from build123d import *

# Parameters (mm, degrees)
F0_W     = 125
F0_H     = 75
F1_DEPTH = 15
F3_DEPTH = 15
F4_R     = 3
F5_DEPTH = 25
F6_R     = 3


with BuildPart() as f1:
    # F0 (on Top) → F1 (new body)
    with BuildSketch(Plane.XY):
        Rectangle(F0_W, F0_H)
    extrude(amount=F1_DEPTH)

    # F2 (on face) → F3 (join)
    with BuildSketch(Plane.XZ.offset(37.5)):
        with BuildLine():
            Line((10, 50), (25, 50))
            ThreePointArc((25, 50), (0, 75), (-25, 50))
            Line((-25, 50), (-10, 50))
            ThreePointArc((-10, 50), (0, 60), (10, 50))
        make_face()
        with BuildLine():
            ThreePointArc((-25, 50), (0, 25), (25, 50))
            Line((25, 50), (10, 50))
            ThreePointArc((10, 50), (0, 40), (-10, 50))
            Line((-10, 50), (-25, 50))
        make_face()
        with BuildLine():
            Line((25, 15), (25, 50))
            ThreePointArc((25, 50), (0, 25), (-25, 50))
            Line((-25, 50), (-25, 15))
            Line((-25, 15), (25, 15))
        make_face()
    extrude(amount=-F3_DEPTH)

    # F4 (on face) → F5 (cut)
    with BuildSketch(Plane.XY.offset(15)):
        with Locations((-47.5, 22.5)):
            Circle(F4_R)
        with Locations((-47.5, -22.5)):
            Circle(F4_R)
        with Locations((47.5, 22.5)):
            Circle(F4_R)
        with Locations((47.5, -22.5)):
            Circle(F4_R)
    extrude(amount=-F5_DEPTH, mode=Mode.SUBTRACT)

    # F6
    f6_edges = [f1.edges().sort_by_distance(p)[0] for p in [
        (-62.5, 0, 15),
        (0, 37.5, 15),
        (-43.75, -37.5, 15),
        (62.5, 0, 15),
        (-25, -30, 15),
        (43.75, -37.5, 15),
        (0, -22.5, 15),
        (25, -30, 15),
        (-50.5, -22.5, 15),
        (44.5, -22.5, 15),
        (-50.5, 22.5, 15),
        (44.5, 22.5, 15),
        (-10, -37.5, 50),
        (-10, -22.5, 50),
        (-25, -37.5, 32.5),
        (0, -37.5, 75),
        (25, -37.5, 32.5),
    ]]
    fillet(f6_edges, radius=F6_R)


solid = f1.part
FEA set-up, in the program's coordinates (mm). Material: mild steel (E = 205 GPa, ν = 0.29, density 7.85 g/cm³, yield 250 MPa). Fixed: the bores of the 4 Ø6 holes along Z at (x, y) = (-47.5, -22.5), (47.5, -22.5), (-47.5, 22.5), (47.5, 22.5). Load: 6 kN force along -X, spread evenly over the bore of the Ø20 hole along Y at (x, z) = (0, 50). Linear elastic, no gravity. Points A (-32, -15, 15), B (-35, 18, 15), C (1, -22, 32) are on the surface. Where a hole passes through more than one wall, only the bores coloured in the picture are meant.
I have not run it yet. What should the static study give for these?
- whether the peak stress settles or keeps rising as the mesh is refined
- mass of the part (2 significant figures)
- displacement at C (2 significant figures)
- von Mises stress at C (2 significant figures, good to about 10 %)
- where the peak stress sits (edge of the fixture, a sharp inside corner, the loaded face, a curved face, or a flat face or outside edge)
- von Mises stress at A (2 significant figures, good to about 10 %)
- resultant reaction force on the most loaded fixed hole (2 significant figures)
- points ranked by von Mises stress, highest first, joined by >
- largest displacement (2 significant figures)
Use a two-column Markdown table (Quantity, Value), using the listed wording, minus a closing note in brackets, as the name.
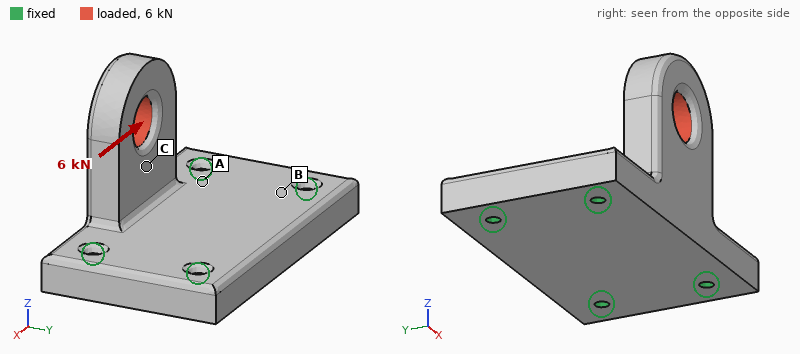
| Quantity | Value |
|---|---|
| whether the peak stress settles or keeps rising as the mesh is refined | keeps rising |
| mass of the part | 1.4 kg |
| displacement at C | 10 µm |
| von Mises stress at C | 34 MPa |
| where the peak stress sits | a sharp inside corner |
| von Mises stress at A | 16 MPa |
| resultant reaction force on the most loaded fixed hole | 4.1 kN |
| points ranked by von Mises stress, highest first, joined by > | C > A > B |
| largest displacement | 32 µm |
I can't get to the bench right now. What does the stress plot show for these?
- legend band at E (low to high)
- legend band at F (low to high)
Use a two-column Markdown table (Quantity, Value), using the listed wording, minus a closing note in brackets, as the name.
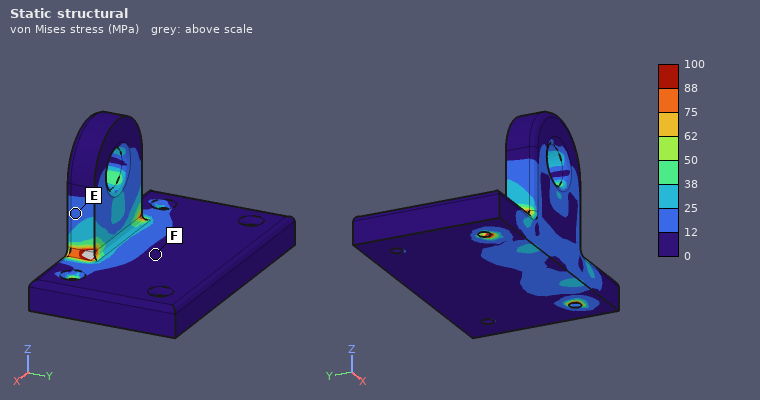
| Quantity | Value |
|---|---|
| legend band at E | 12 to 25 MPa |
| legend band at F | 0 to 12 MPa |
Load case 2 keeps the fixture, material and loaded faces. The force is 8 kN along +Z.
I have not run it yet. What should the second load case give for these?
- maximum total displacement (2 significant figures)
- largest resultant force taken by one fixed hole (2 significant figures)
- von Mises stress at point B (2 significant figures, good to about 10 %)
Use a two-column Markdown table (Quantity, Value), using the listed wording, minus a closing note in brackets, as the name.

| Quantity | Value |
|---|---|
| maximum total displacement | 32 µm |
| largest resultant force taken by one fixed hole | 4.6 kN |
| von Mises stress at point B | 9.4 MPa |
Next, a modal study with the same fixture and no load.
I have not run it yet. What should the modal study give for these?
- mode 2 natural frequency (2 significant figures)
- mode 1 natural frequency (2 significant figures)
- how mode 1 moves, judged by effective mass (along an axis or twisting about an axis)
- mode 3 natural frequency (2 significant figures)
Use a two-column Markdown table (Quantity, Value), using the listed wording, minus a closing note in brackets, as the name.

| Quantity | Value |
|---|---|
| mode 2 natural frequency | 5500 Hz |
| mode 1 natural frequency | 2600 Hz |
| how mode 1 moves, judged by effective mass | along Y |
| mode 3 natural frequency | 5600 Hz |
